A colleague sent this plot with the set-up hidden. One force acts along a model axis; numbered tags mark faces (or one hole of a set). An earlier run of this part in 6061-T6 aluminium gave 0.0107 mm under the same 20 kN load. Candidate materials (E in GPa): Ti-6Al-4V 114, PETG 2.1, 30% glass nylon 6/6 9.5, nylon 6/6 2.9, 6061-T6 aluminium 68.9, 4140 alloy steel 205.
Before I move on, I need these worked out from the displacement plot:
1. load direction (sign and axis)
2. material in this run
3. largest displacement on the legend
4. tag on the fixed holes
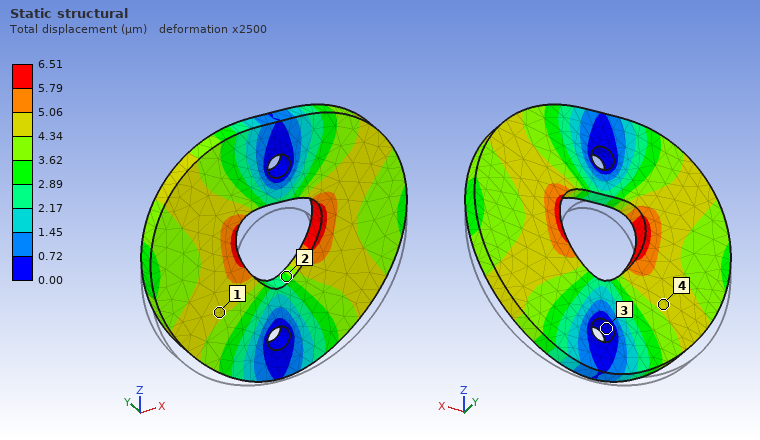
+Z
Ti-6Al-4V
6.51 µm
3
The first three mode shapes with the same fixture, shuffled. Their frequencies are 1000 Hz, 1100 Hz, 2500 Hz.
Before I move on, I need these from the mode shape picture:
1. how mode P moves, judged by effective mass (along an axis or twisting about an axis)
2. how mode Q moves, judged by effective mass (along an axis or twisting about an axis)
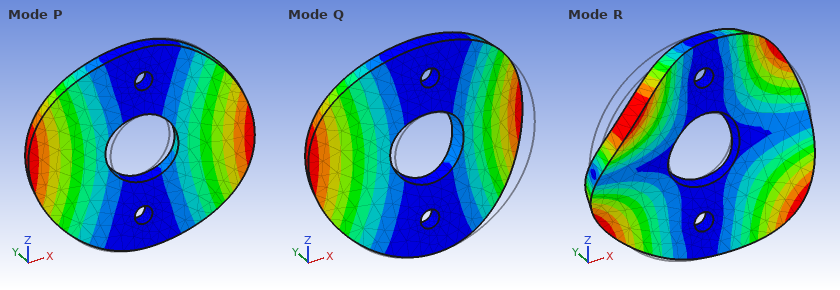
twisting about Z
along Y
